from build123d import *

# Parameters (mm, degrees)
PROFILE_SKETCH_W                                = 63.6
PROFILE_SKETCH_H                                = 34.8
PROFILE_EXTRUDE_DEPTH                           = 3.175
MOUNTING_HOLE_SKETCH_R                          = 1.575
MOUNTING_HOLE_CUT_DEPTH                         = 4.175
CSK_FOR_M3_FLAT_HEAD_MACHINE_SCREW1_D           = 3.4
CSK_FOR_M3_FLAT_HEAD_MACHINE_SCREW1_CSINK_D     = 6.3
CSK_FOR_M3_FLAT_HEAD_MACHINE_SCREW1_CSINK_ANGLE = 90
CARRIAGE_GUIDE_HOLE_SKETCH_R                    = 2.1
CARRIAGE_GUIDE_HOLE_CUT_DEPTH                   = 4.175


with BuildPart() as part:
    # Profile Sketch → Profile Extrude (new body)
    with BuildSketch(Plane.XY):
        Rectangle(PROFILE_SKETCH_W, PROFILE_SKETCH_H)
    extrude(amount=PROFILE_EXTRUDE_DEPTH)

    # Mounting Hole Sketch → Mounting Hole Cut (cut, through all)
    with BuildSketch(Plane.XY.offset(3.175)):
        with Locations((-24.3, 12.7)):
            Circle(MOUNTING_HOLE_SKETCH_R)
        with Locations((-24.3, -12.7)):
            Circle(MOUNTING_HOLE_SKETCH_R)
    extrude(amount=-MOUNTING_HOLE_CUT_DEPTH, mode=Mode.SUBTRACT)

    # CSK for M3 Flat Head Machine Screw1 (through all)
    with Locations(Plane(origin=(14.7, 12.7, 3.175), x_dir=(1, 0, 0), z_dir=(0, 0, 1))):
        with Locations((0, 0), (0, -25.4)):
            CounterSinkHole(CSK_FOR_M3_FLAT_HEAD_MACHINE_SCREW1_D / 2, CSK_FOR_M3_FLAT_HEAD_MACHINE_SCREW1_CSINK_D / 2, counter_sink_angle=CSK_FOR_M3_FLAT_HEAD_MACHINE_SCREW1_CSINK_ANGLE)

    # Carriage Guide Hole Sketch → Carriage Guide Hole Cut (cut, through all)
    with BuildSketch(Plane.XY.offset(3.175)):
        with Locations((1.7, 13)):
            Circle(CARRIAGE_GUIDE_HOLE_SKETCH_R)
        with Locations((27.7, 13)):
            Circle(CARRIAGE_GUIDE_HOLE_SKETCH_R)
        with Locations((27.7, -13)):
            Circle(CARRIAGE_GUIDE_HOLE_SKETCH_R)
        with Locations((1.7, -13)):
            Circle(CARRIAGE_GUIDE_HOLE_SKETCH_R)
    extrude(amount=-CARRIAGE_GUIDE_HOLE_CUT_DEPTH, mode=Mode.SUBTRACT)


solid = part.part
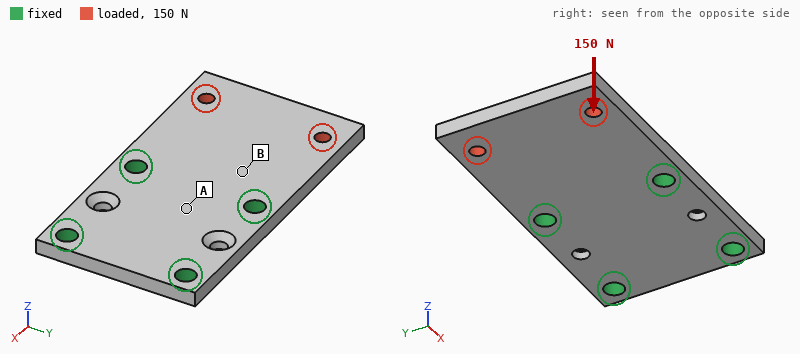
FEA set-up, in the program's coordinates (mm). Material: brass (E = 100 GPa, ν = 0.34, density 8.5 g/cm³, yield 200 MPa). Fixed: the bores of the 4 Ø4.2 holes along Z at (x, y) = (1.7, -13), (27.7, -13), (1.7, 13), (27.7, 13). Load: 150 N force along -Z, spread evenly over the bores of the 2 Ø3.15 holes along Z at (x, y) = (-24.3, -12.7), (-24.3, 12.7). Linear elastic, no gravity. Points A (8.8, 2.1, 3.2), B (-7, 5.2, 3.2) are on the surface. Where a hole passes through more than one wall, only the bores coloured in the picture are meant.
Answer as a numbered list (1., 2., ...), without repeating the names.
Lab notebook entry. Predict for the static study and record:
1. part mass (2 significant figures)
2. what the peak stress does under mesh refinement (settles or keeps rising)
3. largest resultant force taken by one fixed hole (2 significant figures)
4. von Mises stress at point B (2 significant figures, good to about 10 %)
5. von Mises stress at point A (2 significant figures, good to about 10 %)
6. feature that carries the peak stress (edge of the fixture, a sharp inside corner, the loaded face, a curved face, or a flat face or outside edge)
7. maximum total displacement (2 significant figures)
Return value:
1. 57 g
2. keeps rising
3. 89 N
4. 38 MPa
5. 9.3 MPa
6. edge of the fixture
7. 0.13 mm
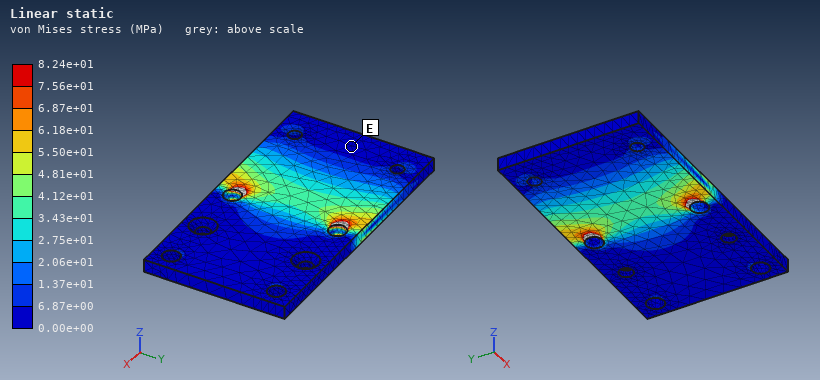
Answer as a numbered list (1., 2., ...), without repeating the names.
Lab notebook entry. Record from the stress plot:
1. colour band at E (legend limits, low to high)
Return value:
1. 0.00e+00 to 6.87e+00 MPa
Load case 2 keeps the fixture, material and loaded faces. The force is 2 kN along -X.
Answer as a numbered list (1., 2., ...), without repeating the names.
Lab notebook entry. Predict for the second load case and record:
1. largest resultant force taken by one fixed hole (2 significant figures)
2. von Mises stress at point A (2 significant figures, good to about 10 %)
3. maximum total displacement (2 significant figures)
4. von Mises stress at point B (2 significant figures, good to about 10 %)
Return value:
1. 900 N
2. 6.7 MPa
3. 7.3 µm
4. 12 MPa
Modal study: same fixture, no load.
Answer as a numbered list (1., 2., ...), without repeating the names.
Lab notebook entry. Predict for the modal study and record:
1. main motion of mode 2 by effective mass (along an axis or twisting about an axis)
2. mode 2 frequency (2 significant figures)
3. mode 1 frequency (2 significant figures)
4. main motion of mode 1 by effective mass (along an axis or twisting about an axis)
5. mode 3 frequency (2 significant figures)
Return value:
1. twisting about X
2. 3900 Hz
3. 1600 Hz
4. along Z
5. 9400 Hz
